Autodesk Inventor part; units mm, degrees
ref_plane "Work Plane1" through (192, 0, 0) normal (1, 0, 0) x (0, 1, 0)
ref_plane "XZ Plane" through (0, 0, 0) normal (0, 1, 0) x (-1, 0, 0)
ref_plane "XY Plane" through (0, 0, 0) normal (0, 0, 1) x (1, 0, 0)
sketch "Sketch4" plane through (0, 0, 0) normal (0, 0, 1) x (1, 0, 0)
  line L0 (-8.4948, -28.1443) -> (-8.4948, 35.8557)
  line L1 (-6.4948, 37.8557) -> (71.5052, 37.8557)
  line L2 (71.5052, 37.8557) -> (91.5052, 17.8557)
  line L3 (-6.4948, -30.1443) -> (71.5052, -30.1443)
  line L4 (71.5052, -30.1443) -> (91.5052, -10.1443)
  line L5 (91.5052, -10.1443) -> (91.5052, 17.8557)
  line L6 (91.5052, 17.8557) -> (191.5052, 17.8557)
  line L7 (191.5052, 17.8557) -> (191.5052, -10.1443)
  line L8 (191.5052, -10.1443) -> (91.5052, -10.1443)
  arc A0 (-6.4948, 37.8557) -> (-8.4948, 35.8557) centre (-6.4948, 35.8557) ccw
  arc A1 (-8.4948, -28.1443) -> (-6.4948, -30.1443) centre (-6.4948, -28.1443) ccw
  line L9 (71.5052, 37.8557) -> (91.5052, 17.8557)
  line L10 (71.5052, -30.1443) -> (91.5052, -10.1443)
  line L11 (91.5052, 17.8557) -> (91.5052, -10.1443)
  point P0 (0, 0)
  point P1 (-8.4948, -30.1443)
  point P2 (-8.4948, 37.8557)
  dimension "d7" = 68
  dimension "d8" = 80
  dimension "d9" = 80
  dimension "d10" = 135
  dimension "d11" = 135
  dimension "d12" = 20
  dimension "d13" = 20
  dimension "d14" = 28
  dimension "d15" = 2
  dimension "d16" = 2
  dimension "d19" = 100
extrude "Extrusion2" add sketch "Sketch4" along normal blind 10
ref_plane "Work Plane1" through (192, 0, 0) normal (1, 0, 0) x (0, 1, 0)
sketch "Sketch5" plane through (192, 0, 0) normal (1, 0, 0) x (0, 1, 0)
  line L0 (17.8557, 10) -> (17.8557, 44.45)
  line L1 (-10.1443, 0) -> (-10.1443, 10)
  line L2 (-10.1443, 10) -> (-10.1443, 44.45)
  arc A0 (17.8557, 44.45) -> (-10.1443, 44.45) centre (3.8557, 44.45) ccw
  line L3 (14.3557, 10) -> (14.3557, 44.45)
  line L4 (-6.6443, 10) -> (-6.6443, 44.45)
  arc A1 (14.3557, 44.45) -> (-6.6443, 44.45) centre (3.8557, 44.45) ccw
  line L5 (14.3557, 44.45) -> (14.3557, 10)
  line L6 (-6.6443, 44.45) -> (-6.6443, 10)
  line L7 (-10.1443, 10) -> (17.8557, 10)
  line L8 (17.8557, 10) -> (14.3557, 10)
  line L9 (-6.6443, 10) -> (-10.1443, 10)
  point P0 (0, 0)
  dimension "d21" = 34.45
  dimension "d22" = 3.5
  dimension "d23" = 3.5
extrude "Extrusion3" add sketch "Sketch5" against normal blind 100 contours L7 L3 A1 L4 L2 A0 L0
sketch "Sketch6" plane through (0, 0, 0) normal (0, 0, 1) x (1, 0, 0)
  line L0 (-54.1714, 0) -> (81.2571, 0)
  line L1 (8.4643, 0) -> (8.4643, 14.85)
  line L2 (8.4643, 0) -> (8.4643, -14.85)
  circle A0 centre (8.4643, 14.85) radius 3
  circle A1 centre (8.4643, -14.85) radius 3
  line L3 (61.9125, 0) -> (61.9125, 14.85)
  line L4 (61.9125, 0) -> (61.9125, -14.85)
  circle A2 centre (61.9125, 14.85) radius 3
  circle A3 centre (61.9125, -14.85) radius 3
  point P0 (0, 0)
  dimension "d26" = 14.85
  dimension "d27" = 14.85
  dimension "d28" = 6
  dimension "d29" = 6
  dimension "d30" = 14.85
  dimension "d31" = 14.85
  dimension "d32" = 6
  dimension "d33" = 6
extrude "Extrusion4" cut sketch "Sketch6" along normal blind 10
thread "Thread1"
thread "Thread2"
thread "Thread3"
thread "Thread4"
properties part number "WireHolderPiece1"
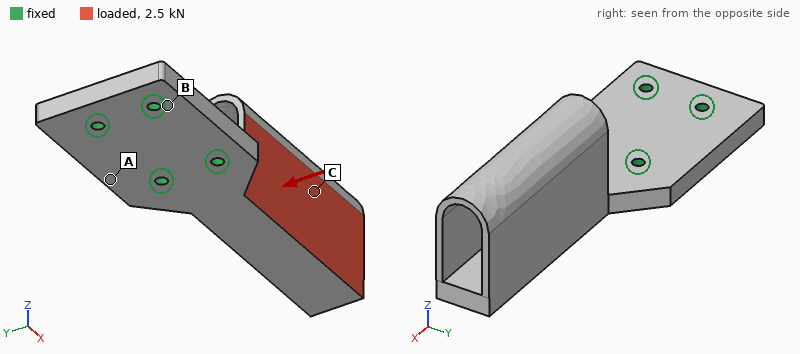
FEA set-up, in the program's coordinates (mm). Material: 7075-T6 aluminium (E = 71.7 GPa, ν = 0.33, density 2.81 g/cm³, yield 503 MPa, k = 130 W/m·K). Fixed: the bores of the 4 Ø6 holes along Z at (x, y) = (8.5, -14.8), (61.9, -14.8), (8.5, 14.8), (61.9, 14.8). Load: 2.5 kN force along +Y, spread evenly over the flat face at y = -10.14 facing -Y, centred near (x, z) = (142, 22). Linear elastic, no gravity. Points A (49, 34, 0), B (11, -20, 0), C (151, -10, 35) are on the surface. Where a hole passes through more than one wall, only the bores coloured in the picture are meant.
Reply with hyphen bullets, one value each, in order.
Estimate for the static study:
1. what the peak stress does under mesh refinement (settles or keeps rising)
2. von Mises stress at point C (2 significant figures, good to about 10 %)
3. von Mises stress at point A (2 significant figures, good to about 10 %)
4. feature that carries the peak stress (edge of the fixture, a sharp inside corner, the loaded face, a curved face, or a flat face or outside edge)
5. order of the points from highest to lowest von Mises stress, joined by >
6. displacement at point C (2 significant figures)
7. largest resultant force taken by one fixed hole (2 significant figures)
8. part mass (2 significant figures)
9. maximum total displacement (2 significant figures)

- keeps rising
- 29 MPa
- 17 MPa
- a sharp inside corner
- C > A > B
- 0.40 mm
- 5.0 kN
- 360 g
- 0.59 mm
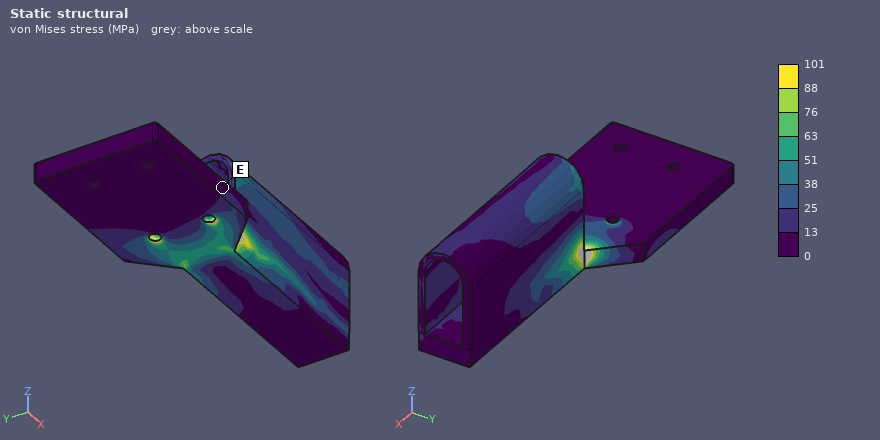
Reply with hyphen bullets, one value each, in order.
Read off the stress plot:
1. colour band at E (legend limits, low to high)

- 0 to 13 MPa
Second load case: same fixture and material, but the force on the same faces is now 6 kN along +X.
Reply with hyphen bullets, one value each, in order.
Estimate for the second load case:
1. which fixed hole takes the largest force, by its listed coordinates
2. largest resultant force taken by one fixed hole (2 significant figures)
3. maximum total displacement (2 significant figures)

- (61.9, -14.8)
- 4.3 kN
- 2.2 mm
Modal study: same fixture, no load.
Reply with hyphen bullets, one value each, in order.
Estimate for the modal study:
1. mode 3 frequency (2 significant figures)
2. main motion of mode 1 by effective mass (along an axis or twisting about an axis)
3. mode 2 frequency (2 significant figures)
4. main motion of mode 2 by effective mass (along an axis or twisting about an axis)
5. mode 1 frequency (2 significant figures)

- 1500 Hz
- along Z
- 940 Hz
- along Y
- 400 Hz
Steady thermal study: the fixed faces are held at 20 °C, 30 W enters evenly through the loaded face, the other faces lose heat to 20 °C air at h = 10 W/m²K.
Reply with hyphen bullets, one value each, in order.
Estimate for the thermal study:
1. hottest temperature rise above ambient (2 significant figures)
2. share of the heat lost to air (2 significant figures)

- 36 K
- 25 %
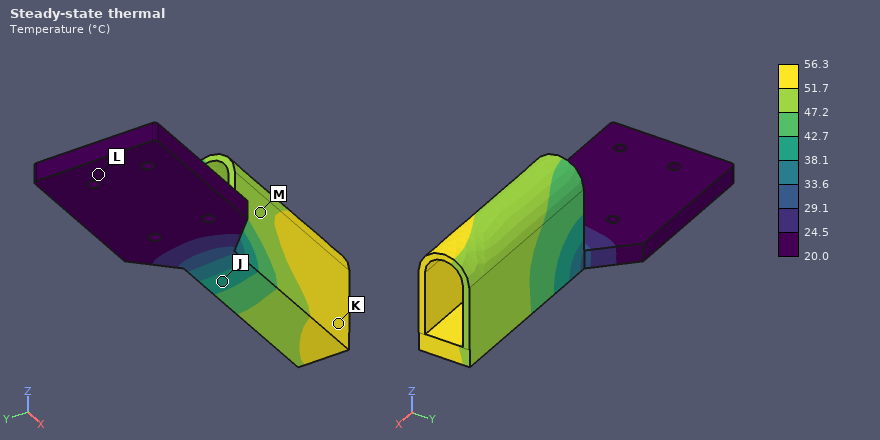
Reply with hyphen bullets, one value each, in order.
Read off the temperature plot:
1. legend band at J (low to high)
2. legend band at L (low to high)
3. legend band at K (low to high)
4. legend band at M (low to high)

- 38.1 to 42.7 °C
- 20.0 to 24.5 °C
- 51.7 to 56.3 °C
- 47.2 to 51.7 °C
